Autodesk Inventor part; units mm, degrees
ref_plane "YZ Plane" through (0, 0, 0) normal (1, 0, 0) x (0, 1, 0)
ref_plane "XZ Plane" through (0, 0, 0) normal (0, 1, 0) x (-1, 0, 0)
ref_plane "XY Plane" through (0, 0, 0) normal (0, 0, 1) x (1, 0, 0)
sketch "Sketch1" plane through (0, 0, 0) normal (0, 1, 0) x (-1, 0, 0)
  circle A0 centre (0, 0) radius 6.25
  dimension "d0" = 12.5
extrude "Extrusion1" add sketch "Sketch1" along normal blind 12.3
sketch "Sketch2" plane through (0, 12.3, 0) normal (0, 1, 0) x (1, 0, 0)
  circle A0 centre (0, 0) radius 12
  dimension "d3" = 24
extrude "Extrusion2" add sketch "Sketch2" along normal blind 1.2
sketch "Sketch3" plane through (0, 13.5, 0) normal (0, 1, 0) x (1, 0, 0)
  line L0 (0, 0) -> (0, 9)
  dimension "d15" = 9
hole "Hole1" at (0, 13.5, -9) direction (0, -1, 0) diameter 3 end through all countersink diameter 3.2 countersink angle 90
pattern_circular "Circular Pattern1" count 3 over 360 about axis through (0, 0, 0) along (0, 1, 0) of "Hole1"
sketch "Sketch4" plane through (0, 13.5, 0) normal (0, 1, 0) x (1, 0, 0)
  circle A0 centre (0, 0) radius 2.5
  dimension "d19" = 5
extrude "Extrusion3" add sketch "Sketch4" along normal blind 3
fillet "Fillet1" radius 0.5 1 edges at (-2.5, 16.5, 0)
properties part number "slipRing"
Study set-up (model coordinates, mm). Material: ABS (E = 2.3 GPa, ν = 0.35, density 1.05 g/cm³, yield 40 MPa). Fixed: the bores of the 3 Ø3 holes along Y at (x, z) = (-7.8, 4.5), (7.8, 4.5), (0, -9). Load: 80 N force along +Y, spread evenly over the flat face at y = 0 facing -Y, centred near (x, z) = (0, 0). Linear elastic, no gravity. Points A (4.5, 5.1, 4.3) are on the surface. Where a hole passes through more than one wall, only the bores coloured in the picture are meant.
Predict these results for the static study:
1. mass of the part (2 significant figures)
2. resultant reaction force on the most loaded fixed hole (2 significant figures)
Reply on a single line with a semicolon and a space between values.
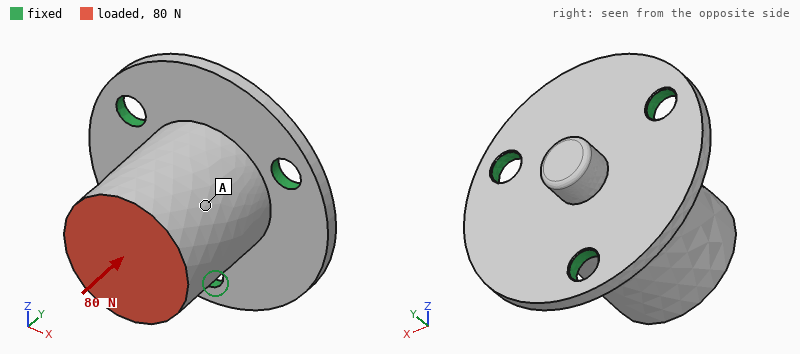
2.2 g; 29 N
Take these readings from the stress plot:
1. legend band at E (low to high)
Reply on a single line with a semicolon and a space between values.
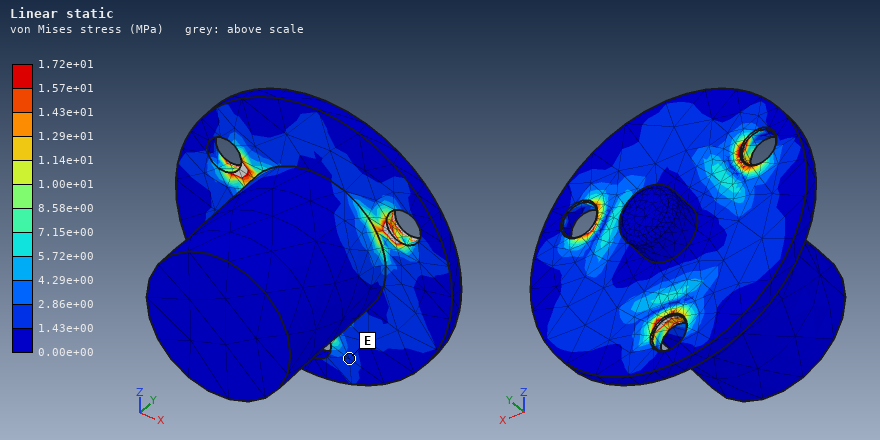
1.43e+00 to 2.86e+00 MPa
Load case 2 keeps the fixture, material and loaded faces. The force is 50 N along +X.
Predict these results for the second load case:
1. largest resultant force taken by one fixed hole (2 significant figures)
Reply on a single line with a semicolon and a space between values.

55 N
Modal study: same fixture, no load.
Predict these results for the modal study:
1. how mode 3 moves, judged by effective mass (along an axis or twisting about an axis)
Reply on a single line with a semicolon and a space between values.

along Y
